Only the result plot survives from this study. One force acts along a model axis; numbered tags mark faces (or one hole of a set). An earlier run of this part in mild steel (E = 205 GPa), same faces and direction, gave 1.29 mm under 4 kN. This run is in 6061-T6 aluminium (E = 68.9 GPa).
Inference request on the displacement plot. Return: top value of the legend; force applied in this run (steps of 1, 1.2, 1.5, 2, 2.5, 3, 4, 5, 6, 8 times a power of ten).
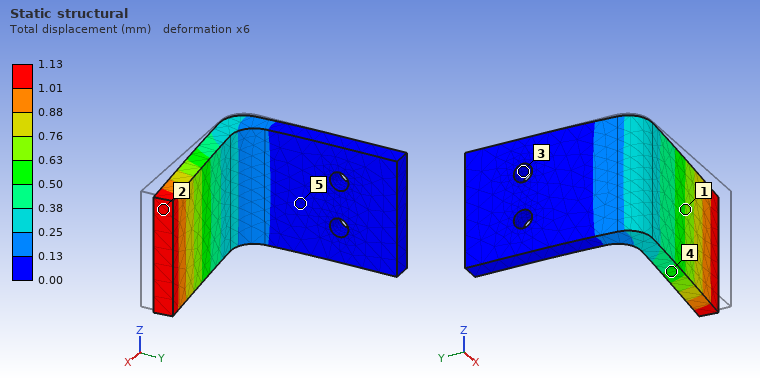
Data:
1.13 mm
1.2 kN
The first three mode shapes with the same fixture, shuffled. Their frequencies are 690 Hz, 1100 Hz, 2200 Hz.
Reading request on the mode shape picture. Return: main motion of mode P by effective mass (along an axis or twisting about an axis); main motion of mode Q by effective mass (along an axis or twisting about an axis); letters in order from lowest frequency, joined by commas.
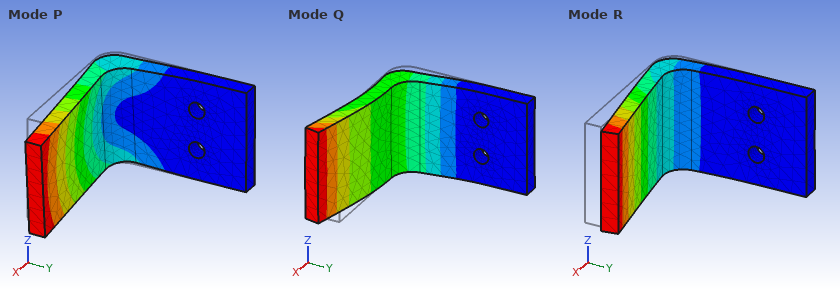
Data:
along Z
along X
R, P, Q
